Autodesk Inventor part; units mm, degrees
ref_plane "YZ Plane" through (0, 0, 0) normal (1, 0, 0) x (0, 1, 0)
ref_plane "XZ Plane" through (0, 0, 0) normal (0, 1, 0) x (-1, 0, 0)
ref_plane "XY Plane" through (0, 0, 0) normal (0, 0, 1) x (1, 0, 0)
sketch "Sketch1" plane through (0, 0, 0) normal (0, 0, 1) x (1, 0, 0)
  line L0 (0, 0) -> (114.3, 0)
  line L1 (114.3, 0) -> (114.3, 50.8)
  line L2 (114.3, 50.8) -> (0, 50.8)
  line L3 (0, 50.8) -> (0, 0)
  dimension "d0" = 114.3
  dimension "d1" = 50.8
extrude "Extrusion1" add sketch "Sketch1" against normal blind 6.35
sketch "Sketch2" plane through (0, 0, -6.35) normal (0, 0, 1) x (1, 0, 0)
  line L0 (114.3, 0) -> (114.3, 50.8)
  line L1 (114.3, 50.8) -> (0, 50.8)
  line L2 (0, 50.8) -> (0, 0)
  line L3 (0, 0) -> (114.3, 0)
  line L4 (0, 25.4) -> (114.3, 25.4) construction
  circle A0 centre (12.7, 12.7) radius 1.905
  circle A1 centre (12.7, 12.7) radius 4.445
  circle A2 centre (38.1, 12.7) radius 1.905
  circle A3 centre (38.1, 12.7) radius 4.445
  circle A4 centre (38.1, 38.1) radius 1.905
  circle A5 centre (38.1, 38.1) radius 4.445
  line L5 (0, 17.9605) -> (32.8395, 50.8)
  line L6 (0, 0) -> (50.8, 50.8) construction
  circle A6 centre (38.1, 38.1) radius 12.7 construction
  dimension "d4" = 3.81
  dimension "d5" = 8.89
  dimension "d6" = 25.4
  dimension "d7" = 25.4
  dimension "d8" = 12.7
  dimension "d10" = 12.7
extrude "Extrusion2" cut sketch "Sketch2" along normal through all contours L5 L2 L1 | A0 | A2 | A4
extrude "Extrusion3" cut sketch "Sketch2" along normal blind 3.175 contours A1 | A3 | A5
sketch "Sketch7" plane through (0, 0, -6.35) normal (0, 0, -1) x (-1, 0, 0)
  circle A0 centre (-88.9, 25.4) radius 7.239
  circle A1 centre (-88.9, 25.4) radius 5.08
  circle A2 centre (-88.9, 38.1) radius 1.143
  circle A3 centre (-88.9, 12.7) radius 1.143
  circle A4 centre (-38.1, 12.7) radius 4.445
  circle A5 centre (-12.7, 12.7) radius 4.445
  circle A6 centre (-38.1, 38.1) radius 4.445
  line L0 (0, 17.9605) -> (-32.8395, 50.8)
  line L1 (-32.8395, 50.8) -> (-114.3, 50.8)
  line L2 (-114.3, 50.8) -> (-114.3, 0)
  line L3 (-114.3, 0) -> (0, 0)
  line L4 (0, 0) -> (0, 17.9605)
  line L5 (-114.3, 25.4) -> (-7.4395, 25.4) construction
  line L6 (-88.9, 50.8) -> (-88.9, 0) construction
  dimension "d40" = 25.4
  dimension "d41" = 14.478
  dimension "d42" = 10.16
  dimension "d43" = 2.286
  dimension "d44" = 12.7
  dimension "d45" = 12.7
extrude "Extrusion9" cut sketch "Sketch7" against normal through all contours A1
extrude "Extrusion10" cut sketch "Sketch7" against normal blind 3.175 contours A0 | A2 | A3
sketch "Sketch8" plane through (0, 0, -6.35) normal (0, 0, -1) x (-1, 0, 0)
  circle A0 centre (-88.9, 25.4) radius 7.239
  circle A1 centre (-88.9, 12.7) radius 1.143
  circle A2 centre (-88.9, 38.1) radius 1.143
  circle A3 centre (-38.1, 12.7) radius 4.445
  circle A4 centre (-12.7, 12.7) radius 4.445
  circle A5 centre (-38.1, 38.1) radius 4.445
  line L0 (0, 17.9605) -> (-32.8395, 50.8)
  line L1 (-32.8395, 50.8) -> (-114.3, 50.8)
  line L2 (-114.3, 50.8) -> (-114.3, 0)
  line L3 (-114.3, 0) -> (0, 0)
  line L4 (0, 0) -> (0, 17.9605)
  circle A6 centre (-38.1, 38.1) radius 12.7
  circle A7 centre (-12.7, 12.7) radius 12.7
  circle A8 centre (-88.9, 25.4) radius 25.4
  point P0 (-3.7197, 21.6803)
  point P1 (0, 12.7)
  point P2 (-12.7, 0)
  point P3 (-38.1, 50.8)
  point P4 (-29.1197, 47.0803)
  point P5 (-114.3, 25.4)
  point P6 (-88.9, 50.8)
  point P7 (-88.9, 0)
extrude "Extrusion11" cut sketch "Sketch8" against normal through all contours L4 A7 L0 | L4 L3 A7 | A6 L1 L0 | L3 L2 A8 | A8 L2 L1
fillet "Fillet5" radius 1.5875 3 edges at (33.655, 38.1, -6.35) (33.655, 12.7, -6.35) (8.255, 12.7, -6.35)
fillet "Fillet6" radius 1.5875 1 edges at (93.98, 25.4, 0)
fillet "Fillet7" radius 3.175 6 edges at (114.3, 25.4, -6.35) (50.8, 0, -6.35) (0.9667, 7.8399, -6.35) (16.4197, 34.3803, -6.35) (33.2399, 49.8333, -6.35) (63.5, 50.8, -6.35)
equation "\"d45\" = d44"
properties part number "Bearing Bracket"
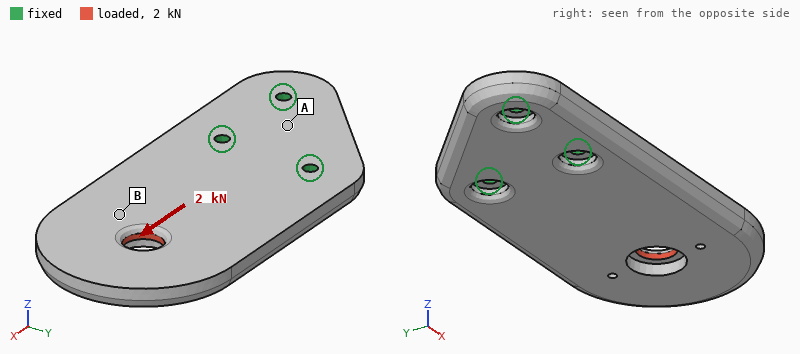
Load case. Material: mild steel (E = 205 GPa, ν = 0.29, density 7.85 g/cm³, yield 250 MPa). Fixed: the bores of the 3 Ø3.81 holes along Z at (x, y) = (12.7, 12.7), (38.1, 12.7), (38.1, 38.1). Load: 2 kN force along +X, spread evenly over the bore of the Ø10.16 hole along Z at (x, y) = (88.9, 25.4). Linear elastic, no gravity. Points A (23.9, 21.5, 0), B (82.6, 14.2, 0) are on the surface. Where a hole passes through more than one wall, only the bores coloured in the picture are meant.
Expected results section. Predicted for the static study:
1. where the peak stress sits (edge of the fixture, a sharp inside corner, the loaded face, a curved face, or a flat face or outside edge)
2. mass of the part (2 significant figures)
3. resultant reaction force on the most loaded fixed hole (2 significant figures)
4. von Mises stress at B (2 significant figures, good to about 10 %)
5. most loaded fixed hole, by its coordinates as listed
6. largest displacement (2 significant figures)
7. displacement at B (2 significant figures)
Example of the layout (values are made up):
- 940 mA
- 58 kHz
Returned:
- the loaded face
- 230 g
- 930 N
- 9.8 MPa
- (38.1, 38.1)
- 12 µm
- 4.3 µm
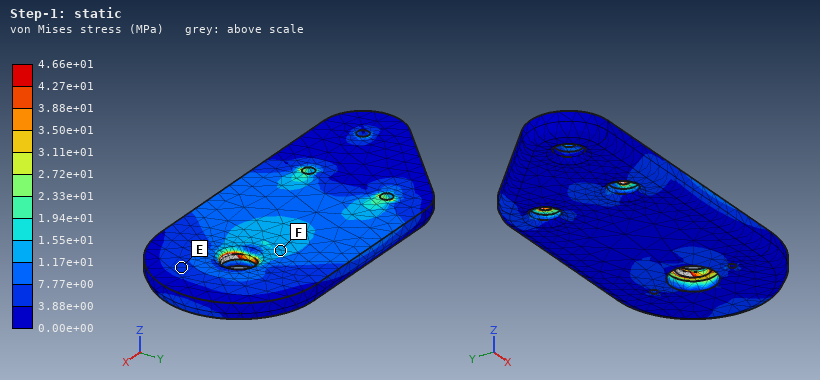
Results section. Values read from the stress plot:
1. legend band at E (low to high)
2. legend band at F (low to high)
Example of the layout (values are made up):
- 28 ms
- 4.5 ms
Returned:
- 3.88e+00 to 7.77e+00 MPa
- 1.17e+01 to 1.55e+01 MPa
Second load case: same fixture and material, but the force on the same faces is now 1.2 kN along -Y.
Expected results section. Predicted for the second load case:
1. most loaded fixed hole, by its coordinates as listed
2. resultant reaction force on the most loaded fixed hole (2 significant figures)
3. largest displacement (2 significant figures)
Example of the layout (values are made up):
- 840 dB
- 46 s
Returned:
- (38.1, 38.1)
- 1.9 kN
- 18 µm
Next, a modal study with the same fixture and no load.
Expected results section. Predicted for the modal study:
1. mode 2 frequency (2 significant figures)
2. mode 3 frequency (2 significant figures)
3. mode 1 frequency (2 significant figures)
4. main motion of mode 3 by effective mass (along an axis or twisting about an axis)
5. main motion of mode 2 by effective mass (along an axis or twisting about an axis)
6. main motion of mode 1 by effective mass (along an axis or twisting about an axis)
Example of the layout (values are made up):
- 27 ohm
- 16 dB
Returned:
- 3100 Hz
- 4900 Hz
- 880 Hz
- along Y
- twisting about X
- along Z
